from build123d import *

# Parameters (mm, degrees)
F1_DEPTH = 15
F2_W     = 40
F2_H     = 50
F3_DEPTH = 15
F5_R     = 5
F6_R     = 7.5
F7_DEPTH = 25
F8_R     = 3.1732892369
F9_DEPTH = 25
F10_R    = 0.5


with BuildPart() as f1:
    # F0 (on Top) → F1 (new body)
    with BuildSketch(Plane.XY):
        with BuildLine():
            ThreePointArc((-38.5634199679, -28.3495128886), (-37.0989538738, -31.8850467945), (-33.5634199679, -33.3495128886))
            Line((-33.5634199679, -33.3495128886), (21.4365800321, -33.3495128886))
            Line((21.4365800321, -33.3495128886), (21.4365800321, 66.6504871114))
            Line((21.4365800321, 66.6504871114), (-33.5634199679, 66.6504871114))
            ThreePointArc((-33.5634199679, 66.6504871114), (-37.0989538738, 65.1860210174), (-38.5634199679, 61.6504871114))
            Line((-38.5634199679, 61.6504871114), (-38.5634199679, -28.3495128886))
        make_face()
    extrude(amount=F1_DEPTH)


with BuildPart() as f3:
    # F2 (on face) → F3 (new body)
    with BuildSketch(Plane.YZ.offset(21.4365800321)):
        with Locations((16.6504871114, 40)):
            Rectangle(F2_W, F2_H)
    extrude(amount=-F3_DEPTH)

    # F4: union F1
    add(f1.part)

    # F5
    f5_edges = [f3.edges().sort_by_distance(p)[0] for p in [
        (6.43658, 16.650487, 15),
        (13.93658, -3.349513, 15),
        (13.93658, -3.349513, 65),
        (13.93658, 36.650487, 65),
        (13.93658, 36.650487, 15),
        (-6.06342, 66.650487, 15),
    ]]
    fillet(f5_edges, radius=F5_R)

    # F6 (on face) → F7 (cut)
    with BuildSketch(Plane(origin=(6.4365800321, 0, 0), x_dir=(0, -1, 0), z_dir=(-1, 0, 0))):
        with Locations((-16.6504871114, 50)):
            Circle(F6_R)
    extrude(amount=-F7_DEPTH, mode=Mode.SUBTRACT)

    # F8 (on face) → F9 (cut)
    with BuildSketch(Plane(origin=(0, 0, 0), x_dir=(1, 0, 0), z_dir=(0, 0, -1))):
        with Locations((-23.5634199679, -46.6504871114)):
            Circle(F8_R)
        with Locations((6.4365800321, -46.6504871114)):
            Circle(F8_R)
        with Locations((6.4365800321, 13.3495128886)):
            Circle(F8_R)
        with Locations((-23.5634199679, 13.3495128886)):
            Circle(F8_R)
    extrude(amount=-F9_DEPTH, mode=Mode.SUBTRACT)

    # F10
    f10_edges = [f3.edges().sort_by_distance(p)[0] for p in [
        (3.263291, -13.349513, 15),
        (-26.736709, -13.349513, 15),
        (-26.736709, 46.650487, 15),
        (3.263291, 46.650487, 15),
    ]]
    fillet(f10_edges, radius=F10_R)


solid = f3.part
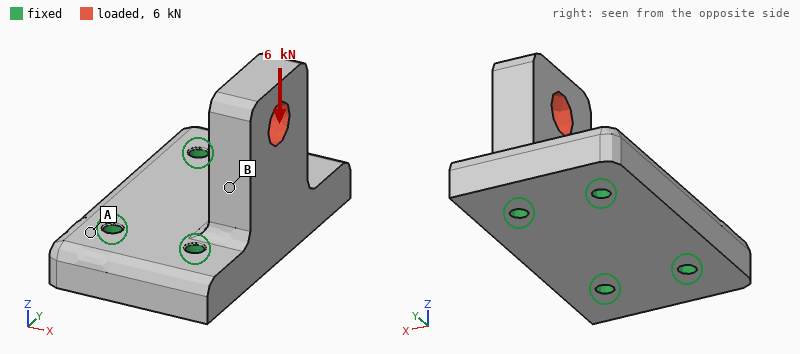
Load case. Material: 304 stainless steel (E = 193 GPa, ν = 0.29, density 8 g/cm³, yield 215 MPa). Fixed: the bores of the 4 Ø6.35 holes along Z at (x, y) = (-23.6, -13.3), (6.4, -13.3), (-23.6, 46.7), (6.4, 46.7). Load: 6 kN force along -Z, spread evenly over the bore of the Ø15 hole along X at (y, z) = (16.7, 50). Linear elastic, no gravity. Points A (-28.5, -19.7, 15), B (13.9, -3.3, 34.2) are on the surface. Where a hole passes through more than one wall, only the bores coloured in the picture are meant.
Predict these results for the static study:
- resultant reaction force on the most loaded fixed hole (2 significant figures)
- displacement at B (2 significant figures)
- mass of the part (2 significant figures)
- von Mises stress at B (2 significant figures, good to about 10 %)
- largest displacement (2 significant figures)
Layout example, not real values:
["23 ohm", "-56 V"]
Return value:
["3.3 kN", "6.7 µm", "920 g", "10 MPa", "13 µm"]
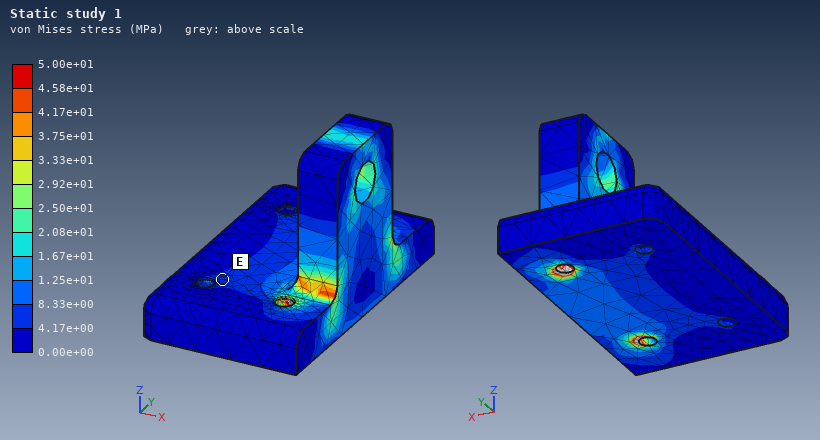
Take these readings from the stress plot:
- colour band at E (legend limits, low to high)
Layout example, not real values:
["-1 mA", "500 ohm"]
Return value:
["4.17e+00 to 8.33e+00 MPa"]
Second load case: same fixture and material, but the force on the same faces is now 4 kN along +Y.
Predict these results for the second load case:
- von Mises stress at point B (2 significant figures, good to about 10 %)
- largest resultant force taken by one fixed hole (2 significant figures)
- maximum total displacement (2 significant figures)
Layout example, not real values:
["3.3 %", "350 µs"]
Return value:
["19 MPa", "3.6 kN", "20 µm"]
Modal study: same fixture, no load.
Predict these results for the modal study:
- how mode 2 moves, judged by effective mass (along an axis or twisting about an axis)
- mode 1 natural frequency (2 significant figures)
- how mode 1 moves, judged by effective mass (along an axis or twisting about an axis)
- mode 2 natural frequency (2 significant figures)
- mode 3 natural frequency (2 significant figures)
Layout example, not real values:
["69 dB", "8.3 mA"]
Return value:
["along Y", "3500 Hz", "along X", "7000 Hz", "9300 Hz"]
